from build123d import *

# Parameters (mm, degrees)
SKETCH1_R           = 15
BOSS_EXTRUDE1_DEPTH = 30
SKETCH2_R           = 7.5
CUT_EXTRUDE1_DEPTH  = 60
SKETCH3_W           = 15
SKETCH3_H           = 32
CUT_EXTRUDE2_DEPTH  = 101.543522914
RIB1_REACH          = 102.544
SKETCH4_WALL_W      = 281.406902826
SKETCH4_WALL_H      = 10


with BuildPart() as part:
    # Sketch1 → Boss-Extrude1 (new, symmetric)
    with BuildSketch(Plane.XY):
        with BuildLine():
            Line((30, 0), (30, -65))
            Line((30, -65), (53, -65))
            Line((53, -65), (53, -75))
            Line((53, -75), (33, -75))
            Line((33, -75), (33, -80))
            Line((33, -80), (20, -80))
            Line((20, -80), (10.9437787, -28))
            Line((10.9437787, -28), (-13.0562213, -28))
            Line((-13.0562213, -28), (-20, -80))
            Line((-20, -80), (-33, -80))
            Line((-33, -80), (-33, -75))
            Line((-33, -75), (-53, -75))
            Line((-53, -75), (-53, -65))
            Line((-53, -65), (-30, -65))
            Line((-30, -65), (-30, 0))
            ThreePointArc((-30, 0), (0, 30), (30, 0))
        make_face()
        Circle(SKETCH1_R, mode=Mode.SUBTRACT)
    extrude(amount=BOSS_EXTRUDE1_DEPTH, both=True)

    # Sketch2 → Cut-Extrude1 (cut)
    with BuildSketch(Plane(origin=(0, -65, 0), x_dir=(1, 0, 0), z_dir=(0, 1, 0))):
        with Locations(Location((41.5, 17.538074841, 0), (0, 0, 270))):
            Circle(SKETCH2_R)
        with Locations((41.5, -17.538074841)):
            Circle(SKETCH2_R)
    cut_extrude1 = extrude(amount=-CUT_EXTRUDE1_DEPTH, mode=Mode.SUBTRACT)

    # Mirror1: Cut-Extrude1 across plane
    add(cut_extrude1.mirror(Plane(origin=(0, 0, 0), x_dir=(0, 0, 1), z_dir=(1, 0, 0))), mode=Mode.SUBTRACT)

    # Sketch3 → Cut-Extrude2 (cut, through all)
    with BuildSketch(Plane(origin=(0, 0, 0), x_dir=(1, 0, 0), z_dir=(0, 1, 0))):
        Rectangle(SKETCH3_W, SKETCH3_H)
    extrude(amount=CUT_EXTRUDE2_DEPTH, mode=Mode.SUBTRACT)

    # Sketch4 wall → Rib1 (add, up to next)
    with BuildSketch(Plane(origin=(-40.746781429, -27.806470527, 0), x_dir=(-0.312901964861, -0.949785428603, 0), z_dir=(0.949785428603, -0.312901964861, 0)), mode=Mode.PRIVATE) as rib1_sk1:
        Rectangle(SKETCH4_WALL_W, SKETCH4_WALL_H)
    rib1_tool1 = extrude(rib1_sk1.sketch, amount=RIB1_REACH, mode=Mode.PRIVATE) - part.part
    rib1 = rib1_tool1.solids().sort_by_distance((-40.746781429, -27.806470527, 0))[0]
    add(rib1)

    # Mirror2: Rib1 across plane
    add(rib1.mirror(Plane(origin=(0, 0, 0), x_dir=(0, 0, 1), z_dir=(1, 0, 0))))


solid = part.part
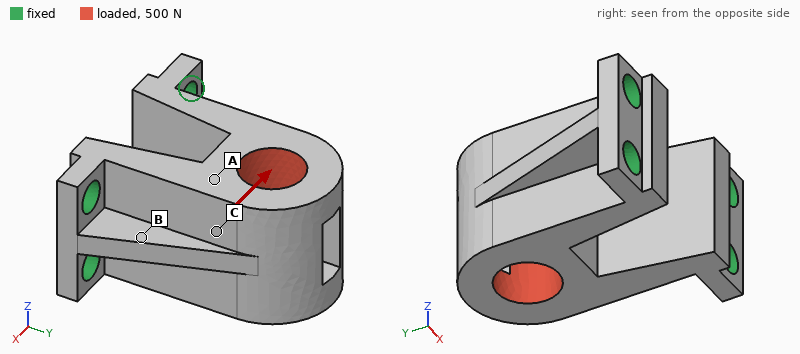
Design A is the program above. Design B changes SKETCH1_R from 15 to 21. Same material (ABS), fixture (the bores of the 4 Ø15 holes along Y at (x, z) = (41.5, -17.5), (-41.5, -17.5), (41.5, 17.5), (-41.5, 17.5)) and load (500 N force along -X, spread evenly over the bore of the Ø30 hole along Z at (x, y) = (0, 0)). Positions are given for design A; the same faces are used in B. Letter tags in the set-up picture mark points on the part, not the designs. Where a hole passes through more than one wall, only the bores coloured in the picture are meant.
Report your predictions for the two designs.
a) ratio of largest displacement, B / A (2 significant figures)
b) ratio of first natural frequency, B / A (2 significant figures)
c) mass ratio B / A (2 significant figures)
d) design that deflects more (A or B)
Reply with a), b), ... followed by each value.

a) 1.9
b) 1.2
c) 0.86
d) B
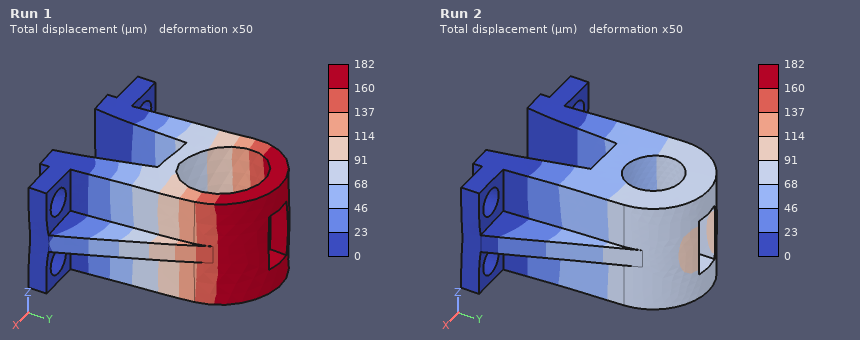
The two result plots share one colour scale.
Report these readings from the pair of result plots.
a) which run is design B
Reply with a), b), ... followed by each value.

a) Run 1
